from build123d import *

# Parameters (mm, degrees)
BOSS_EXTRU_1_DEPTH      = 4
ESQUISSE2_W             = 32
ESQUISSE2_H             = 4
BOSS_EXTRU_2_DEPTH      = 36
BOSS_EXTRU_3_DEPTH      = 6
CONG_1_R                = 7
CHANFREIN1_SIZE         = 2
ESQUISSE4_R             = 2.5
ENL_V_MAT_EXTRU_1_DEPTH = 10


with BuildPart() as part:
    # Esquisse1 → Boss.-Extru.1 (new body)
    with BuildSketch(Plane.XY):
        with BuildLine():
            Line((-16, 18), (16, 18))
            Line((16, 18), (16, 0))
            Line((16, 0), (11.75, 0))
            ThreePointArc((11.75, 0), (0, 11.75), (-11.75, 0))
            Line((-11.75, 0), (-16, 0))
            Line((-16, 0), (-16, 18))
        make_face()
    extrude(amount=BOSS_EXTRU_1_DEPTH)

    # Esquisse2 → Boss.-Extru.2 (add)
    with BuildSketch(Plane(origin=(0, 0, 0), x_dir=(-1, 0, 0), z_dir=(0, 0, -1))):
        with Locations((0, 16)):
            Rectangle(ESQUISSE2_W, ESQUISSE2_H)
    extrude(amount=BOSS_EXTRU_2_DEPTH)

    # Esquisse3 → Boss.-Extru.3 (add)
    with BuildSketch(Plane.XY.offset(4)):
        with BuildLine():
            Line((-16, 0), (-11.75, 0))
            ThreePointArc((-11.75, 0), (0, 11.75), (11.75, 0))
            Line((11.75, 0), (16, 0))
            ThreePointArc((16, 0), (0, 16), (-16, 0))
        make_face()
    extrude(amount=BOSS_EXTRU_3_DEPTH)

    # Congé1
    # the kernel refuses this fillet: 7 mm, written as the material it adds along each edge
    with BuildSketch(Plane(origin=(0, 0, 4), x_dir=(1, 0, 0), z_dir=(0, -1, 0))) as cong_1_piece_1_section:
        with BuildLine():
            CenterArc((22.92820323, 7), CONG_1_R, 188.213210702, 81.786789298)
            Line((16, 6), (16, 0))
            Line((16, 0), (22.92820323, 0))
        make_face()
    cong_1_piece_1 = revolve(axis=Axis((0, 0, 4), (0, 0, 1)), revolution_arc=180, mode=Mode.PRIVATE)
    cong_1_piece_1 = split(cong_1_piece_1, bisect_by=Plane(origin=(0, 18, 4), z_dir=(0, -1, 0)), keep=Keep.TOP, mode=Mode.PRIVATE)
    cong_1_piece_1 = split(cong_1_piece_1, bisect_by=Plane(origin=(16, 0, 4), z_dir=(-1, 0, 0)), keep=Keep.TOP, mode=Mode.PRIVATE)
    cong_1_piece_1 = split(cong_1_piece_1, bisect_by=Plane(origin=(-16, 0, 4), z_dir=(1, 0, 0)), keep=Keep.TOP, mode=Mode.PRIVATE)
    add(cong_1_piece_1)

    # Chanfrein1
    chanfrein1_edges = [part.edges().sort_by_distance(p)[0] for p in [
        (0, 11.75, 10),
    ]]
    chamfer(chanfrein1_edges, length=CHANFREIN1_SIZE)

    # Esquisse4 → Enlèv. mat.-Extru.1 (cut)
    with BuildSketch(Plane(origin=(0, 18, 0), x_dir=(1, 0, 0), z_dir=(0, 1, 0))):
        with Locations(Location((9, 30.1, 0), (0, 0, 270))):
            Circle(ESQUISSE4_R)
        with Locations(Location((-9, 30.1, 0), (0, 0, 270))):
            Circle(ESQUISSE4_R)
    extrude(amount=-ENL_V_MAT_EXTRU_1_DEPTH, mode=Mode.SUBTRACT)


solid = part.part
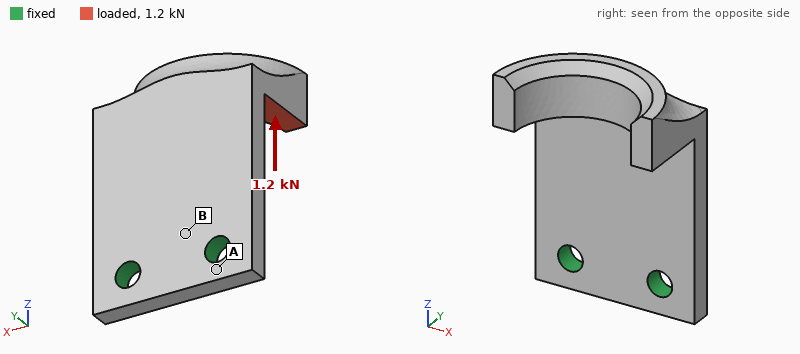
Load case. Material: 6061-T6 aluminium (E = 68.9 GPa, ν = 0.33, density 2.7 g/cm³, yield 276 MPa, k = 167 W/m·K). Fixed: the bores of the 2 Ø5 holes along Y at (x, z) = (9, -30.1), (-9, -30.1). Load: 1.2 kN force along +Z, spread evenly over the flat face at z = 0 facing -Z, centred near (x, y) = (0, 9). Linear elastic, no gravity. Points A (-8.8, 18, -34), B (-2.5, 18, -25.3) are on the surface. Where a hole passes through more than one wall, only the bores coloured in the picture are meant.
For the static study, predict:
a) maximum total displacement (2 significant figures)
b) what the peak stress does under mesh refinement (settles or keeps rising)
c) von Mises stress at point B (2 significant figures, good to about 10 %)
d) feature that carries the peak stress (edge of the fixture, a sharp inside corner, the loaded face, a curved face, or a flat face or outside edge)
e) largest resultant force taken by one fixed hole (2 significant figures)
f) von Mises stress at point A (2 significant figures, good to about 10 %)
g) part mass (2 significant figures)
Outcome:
0.62 mm
keeps rising
74 MPa
edge of the fixture
610 N
15 MPa
20 g
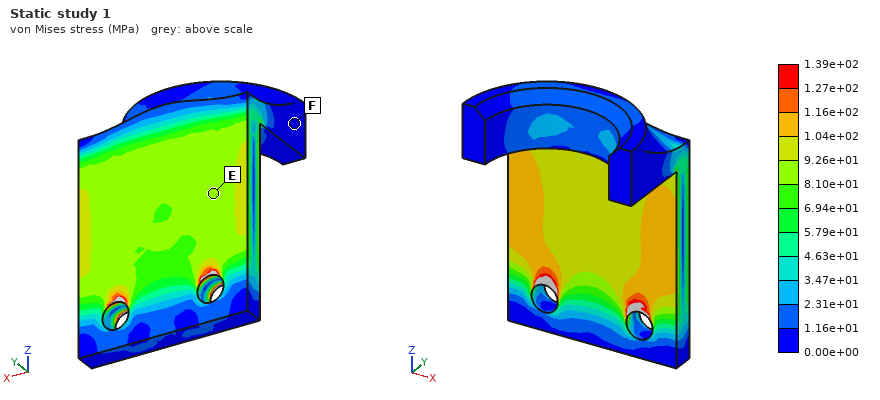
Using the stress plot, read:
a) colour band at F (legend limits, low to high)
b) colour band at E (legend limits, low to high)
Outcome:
0.00e+00 to 1.16e+01 MPa
8.10e+01 to 9.26e+01 MPa
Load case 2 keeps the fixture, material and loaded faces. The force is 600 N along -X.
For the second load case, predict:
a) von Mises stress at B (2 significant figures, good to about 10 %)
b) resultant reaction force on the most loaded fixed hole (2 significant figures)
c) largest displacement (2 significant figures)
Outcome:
10 MPa
900 N
0.13 mm
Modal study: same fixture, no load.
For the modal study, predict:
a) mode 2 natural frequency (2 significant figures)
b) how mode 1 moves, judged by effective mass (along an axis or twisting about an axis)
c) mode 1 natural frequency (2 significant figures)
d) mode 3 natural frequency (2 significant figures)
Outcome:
3800 Hz
along Y
1600 Hz
8200 Hz
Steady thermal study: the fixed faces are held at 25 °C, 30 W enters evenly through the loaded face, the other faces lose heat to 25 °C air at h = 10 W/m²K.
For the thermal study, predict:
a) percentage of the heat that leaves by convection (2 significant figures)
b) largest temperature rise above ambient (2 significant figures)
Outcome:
3.4 %
53 K
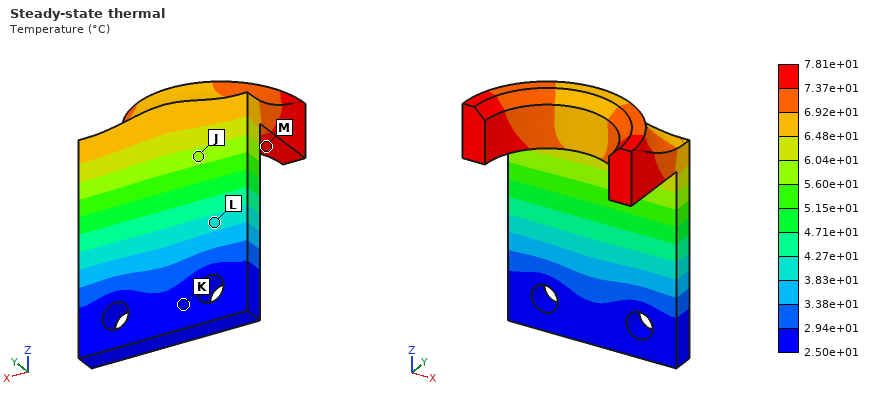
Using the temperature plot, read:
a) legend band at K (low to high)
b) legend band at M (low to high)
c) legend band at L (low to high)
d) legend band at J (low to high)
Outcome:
2.50e+01 to 2.94e+01 °C
7.37e+01 to 7.81e+01 °C
3.83e+01 to 4.27e+01 °C
5.60e+01 to 6.04e+01 °C
